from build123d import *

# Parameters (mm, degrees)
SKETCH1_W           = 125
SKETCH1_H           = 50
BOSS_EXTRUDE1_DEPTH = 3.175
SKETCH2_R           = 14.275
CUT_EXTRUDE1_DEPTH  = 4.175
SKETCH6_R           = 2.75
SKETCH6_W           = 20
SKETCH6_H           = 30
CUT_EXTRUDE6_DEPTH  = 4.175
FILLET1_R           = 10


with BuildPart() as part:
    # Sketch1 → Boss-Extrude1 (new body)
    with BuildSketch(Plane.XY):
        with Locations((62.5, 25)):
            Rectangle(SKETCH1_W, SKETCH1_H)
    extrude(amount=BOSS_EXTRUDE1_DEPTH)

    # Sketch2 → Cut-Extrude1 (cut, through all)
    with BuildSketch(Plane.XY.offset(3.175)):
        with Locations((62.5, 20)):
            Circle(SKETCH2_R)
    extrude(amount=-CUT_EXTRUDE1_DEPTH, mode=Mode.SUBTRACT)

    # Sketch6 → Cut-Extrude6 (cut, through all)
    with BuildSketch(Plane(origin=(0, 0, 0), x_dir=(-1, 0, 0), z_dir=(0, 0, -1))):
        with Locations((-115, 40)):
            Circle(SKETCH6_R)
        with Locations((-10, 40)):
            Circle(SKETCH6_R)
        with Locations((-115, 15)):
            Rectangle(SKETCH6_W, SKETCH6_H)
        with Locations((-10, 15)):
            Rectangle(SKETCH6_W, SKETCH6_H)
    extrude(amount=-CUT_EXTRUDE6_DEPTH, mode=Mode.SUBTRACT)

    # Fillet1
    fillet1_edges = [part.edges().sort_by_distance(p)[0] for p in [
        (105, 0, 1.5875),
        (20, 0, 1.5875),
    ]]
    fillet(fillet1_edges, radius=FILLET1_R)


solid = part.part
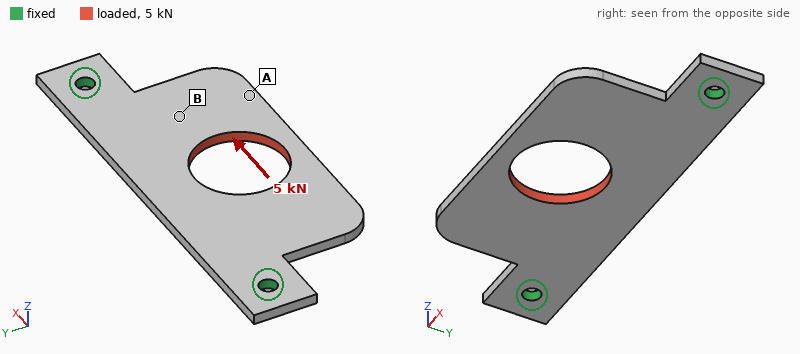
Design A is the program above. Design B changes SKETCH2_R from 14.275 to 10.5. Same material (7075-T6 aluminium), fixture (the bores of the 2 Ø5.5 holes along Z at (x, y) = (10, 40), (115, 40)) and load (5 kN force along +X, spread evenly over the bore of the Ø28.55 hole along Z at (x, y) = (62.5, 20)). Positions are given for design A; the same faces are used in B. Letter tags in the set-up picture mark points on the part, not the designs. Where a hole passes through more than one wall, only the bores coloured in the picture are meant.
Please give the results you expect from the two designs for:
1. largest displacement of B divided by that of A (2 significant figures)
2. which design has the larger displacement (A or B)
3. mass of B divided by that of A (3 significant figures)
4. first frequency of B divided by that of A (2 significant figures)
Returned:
0.76
A
1.07
0.96
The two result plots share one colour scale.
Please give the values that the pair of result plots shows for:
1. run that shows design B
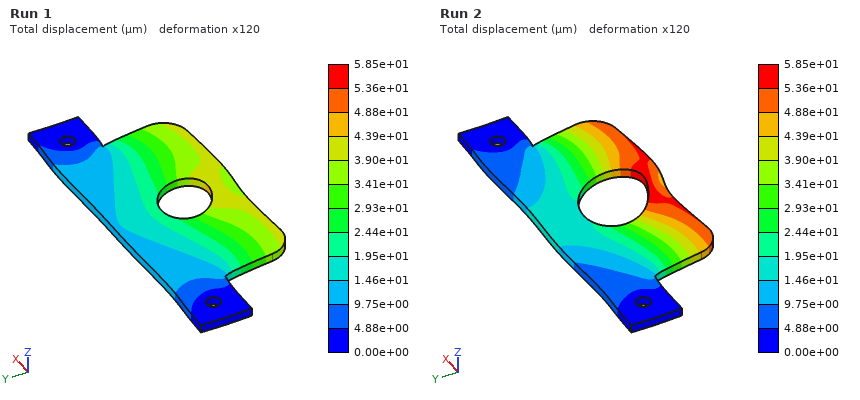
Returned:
Run 1
